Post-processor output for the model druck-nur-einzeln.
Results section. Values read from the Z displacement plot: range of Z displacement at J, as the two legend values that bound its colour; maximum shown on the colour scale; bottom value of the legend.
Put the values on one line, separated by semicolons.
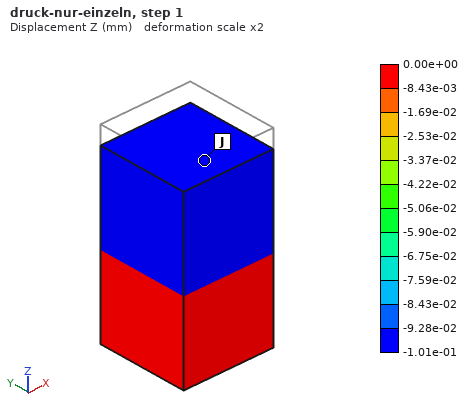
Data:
-1.01e-01 to -9.28e-02 mm; 0.00e+00 mm; -1.01e-01 mm
